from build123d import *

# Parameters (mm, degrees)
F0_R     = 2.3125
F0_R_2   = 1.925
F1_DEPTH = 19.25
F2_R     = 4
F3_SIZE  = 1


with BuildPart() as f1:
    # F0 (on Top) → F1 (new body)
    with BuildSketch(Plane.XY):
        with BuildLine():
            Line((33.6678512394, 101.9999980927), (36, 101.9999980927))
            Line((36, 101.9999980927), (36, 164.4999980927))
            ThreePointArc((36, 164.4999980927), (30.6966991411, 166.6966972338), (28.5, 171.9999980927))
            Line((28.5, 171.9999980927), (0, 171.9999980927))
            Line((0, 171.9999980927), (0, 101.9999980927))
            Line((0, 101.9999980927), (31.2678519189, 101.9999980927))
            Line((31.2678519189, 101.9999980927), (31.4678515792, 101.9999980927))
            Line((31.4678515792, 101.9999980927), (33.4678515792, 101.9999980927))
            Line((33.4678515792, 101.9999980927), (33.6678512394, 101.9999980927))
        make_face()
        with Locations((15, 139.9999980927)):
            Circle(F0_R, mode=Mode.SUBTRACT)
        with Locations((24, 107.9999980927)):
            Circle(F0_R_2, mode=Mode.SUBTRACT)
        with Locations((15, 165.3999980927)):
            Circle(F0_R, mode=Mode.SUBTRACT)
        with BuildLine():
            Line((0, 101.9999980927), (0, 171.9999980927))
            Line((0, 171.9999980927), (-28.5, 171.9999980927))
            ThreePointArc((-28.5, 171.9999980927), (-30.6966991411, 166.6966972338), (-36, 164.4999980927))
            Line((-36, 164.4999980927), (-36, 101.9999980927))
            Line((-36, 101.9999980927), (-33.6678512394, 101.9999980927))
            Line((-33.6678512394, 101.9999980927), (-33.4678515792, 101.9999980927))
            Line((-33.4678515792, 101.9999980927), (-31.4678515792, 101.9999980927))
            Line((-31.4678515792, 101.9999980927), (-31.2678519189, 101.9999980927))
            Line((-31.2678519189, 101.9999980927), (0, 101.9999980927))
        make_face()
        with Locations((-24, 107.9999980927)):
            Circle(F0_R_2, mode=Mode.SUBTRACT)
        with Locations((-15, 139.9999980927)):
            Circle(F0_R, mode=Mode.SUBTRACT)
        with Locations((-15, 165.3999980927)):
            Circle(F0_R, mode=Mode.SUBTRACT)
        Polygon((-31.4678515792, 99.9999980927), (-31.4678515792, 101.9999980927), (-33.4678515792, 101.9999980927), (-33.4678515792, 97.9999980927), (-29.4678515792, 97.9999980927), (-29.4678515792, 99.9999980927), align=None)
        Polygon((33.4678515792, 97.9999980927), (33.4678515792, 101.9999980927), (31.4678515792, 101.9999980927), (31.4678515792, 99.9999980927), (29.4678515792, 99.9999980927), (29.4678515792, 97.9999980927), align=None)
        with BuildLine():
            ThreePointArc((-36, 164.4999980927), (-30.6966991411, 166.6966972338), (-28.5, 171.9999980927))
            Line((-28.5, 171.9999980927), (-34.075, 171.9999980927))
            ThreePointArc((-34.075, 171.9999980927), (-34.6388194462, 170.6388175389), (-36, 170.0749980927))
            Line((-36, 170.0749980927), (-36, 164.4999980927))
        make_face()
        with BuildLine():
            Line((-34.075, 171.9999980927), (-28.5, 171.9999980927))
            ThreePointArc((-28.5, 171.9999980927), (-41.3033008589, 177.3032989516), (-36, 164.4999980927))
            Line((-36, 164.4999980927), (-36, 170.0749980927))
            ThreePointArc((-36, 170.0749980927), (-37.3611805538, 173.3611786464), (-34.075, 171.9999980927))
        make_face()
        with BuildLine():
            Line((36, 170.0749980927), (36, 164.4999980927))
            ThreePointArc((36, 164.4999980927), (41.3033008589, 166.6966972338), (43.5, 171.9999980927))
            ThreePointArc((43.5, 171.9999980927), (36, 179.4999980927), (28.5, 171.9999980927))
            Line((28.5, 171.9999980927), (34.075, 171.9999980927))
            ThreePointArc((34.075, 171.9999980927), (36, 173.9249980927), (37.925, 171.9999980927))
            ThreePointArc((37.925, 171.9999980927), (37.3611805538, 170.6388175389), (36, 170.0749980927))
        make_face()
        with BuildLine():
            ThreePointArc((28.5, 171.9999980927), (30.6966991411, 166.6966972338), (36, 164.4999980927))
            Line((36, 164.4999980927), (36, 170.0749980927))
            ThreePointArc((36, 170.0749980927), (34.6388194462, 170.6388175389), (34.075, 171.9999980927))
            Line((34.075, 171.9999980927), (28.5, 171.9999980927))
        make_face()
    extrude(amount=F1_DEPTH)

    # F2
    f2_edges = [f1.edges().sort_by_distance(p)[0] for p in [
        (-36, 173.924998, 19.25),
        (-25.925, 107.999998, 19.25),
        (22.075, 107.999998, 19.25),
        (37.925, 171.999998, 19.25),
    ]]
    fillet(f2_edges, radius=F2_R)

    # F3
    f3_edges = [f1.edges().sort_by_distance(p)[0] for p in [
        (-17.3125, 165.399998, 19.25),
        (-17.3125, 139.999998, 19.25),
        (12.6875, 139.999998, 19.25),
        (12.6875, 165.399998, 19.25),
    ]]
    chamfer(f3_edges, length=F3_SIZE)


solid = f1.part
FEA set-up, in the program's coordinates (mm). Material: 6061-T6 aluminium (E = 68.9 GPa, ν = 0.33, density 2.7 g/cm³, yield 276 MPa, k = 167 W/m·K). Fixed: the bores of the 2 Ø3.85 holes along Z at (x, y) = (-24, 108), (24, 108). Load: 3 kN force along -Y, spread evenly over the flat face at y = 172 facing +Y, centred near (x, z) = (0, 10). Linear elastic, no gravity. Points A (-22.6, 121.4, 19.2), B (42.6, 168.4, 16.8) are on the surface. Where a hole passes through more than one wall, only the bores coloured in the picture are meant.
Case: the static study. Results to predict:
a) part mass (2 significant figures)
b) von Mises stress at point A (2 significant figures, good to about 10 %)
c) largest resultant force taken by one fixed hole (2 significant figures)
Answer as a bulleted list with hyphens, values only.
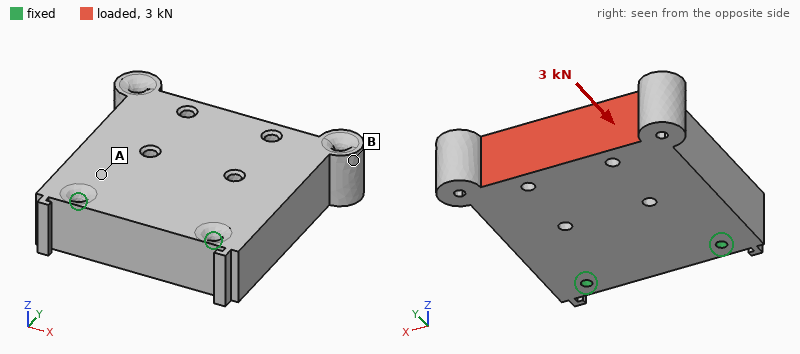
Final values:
- 270 g
- 3.3 MPa
- 1.5 kN
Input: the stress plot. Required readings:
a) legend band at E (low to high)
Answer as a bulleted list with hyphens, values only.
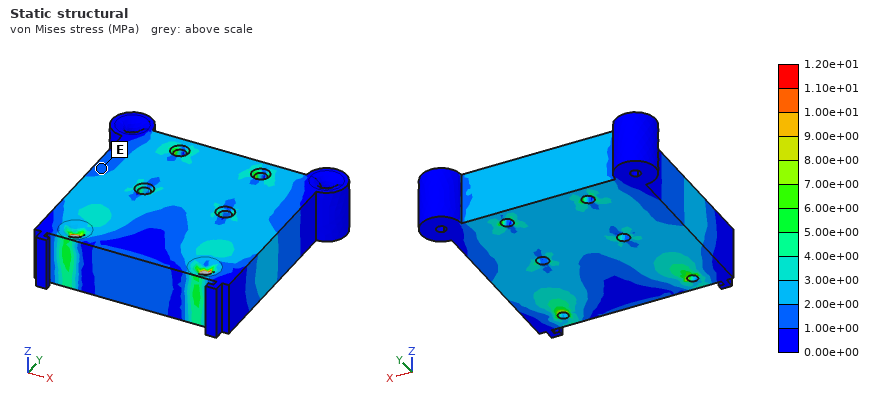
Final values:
- 1.00e+00 to 2.00e+00 MPa
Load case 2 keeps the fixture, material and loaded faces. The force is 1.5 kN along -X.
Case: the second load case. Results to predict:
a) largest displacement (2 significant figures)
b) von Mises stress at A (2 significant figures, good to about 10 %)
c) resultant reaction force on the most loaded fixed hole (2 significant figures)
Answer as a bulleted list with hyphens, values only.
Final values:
- 11 µm
- 3.6 MPa
- 2.1 kN
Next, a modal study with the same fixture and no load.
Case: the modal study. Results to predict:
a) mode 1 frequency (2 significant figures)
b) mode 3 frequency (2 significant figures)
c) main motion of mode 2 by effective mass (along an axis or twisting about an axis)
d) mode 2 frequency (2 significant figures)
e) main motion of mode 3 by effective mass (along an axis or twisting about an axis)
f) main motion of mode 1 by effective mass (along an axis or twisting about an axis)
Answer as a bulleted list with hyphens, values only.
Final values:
- 2300 Hz
- 6400 Hz
- twisting about Y
- 5200 Hz
- along X
- along Z
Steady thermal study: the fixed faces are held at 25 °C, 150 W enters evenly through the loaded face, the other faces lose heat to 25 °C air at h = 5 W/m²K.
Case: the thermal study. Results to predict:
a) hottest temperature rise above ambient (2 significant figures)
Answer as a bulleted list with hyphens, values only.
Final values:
- 51 K
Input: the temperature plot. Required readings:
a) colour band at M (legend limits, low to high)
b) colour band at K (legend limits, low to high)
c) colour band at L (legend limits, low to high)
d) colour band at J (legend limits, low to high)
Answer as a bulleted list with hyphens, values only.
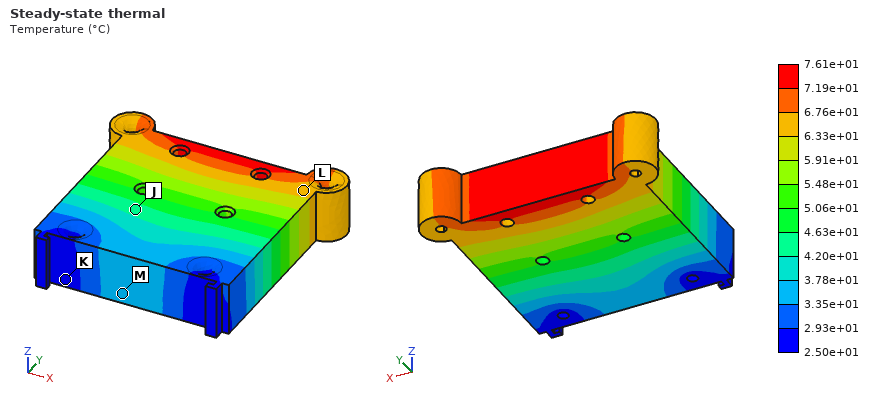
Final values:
- 3.35e+01 to 3.78e+01 °C
- 2.50e+01 to 2.93e+01 °C
- 6.33e+01 to 6.76e+01 °C
- 4.20e+01 to 4.63e+01 °C
